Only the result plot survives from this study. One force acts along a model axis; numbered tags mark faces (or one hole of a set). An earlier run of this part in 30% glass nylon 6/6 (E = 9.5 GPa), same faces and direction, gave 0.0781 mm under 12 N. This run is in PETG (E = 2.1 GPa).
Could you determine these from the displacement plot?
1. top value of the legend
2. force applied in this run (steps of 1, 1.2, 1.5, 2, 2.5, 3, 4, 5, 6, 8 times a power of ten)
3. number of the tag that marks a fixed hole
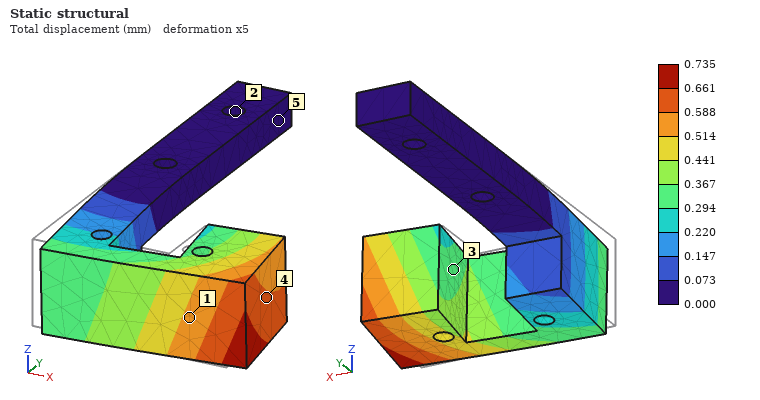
0.735 mm
25 N
2
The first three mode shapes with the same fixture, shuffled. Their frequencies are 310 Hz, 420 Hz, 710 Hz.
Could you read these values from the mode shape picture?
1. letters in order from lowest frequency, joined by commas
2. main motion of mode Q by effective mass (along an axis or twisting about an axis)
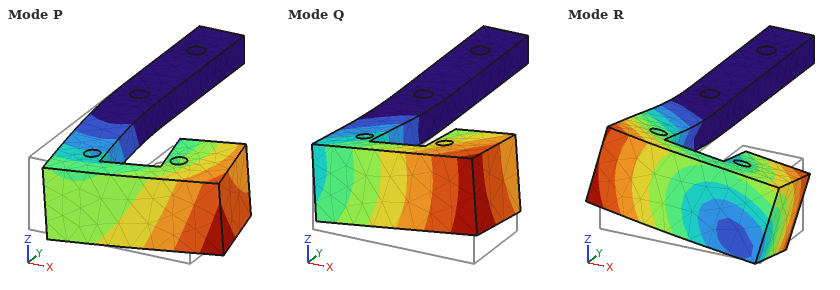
Q, P, R
along Z
